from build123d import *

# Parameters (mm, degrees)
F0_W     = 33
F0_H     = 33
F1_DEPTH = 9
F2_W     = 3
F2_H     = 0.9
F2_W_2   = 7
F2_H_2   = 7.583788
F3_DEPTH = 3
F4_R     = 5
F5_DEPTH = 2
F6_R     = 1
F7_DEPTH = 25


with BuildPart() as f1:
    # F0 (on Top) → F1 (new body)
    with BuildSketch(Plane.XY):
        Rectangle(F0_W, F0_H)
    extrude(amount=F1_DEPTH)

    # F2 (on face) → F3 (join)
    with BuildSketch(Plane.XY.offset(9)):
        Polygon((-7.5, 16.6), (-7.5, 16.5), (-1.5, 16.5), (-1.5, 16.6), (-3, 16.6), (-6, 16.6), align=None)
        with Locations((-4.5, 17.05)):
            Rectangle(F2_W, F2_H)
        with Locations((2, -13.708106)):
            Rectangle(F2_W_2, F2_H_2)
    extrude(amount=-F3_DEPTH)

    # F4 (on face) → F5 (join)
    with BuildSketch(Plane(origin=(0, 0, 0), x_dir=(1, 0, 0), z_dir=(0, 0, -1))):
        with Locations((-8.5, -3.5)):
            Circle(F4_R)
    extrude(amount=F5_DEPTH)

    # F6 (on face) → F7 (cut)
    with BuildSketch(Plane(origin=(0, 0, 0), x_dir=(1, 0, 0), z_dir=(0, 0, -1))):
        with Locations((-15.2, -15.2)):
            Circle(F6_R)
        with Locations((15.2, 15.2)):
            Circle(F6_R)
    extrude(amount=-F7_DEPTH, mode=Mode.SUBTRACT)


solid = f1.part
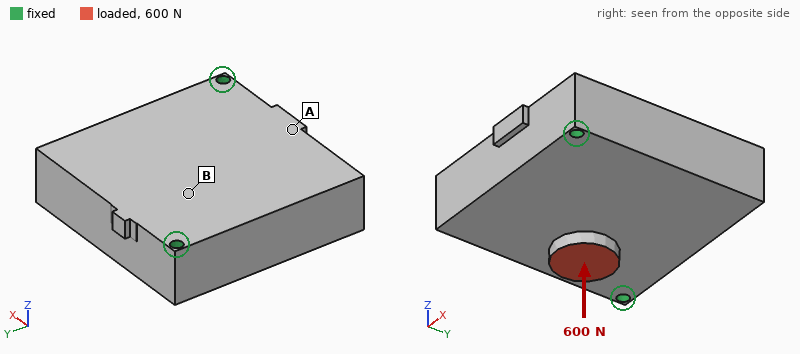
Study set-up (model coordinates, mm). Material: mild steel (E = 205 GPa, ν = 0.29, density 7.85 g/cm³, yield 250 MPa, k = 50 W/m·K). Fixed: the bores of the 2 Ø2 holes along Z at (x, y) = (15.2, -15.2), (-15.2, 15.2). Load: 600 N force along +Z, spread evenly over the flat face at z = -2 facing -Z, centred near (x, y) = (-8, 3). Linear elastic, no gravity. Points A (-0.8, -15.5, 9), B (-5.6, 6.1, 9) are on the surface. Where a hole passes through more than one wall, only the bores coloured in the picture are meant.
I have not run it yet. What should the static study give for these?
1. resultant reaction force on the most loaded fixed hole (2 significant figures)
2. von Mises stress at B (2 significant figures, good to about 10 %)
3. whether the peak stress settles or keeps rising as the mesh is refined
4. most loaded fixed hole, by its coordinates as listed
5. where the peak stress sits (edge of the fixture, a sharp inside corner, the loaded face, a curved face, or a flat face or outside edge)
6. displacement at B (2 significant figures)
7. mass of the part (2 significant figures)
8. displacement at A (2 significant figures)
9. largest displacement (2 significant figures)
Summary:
440 N
8.4 MPa
keeps rising
(-15.2, 15.2)
edge of the fixture
1.5 µm
78 g
2.3 µm
4.6 µm
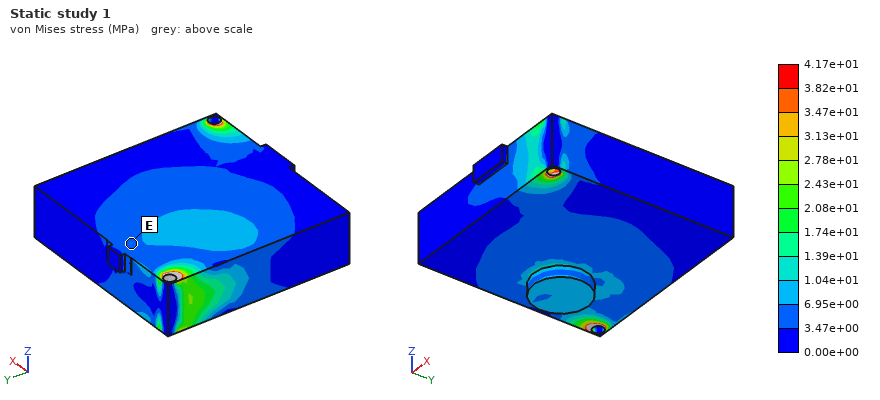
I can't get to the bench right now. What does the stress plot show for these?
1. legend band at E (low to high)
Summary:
3.47e+00 to 6.95e+00 MPa
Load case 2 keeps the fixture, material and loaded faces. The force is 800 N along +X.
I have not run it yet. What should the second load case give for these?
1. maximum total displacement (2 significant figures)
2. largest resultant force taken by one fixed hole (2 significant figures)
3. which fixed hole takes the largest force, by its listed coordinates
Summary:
5.2 µm
500 N
(-15.2, 15.2)
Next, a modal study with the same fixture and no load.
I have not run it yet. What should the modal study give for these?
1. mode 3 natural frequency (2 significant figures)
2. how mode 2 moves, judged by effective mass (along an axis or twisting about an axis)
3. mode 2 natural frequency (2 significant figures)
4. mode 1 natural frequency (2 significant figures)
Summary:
18 kHz
along Z
11 kHz
7500 Hz
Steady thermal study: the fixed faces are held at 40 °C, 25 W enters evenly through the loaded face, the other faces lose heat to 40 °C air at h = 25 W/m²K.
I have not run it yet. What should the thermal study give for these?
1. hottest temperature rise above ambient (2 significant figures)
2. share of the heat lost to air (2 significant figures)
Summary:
62 K
8.4 %
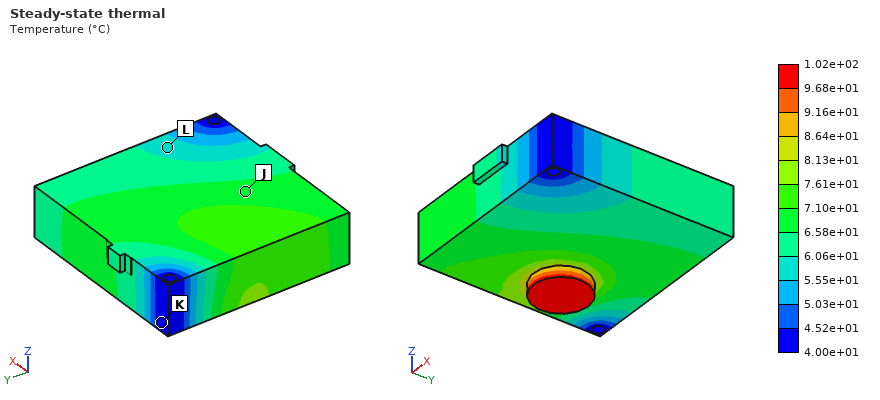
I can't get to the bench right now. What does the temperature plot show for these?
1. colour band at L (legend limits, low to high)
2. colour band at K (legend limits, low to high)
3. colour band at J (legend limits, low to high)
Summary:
5.55e+01 to 6.06e+01 °C
4.00e+01 to 4.52e+01 °C
6.58e+01 to 7.10e+01 °C
